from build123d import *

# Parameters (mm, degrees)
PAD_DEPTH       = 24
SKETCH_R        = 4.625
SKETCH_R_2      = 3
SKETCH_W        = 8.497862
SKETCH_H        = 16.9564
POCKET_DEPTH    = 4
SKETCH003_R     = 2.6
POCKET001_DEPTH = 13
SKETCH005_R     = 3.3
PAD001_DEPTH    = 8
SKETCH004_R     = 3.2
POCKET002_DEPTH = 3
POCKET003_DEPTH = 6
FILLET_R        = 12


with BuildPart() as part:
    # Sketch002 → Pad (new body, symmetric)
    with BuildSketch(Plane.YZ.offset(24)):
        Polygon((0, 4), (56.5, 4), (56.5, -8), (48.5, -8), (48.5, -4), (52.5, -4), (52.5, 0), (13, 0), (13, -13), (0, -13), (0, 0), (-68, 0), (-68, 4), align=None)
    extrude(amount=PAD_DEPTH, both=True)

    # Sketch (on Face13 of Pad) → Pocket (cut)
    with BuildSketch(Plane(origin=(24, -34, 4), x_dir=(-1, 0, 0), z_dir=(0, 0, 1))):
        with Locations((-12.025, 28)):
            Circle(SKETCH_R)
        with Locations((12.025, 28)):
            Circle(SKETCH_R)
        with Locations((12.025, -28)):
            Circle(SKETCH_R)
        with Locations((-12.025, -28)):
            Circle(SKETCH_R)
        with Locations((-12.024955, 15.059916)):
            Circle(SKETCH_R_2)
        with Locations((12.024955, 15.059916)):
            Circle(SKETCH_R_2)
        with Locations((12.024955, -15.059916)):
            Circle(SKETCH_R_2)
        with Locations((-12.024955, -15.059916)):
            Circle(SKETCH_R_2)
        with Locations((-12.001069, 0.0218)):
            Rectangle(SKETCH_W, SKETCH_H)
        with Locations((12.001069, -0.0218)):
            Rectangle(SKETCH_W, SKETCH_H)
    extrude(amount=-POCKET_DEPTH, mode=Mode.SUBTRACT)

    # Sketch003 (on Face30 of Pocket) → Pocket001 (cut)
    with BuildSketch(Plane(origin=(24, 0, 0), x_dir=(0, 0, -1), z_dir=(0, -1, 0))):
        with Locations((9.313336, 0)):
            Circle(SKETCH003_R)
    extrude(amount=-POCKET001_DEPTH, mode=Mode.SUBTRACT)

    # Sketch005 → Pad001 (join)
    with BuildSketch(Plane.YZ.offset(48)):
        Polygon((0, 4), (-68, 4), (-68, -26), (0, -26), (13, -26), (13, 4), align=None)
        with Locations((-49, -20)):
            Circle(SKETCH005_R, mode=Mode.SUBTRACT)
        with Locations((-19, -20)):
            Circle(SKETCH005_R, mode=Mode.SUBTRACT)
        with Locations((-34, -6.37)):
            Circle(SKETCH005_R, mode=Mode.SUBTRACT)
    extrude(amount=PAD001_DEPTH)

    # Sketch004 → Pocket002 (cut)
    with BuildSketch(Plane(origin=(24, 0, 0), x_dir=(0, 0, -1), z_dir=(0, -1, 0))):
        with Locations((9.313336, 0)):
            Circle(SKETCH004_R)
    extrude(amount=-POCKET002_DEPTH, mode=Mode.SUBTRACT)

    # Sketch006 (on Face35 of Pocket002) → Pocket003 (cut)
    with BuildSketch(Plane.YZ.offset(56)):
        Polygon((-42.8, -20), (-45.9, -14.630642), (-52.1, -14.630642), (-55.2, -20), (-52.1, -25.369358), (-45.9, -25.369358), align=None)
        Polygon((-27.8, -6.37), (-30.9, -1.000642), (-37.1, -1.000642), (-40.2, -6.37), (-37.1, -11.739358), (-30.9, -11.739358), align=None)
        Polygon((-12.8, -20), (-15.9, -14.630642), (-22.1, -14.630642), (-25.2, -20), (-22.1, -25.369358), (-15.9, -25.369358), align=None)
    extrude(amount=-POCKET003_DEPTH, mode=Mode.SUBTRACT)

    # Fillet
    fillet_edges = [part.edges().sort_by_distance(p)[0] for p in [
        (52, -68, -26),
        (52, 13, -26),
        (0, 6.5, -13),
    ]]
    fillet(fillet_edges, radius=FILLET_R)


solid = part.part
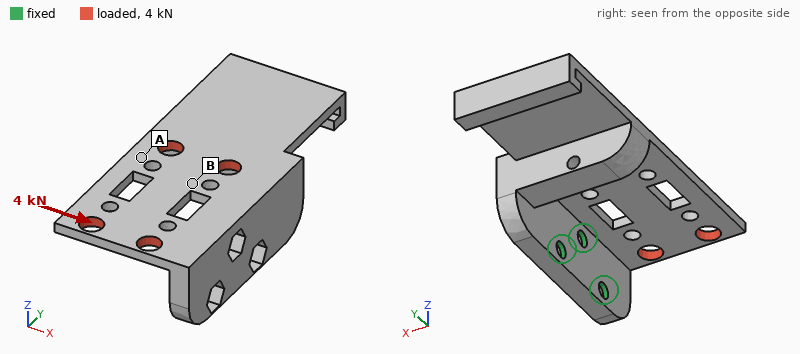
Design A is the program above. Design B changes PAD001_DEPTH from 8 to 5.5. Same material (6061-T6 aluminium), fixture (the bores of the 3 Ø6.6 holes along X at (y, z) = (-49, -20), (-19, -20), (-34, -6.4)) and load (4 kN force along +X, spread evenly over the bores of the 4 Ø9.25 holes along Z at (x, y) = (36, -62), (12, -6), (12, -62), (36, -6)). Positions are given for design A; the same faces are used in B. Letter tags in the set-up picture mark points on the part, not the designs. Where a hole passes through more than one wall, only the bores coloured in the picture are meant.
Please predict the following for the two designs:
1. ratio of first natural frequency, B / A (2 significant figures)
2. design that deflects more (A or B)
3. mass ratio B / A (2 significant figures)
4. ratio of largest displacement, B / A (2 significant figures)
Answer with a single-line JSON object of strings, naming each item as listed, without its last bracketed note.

{"ratio of first natural frequency, B / A": "0.77", "design that deflects more": "B", "mass ratio B / A": "0.89", "ratio of largest displacement, B / A": "1.6"}
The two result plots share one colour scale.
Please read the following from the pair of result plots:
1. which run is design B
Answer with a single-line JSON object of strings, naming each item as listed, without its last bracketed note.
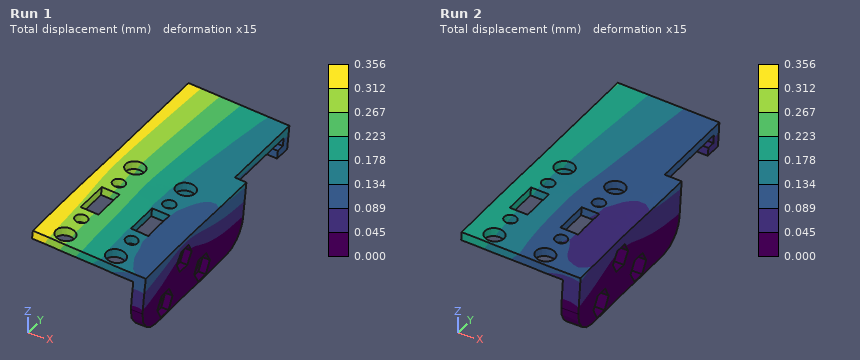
{"which run is design B": "Run 1"}
